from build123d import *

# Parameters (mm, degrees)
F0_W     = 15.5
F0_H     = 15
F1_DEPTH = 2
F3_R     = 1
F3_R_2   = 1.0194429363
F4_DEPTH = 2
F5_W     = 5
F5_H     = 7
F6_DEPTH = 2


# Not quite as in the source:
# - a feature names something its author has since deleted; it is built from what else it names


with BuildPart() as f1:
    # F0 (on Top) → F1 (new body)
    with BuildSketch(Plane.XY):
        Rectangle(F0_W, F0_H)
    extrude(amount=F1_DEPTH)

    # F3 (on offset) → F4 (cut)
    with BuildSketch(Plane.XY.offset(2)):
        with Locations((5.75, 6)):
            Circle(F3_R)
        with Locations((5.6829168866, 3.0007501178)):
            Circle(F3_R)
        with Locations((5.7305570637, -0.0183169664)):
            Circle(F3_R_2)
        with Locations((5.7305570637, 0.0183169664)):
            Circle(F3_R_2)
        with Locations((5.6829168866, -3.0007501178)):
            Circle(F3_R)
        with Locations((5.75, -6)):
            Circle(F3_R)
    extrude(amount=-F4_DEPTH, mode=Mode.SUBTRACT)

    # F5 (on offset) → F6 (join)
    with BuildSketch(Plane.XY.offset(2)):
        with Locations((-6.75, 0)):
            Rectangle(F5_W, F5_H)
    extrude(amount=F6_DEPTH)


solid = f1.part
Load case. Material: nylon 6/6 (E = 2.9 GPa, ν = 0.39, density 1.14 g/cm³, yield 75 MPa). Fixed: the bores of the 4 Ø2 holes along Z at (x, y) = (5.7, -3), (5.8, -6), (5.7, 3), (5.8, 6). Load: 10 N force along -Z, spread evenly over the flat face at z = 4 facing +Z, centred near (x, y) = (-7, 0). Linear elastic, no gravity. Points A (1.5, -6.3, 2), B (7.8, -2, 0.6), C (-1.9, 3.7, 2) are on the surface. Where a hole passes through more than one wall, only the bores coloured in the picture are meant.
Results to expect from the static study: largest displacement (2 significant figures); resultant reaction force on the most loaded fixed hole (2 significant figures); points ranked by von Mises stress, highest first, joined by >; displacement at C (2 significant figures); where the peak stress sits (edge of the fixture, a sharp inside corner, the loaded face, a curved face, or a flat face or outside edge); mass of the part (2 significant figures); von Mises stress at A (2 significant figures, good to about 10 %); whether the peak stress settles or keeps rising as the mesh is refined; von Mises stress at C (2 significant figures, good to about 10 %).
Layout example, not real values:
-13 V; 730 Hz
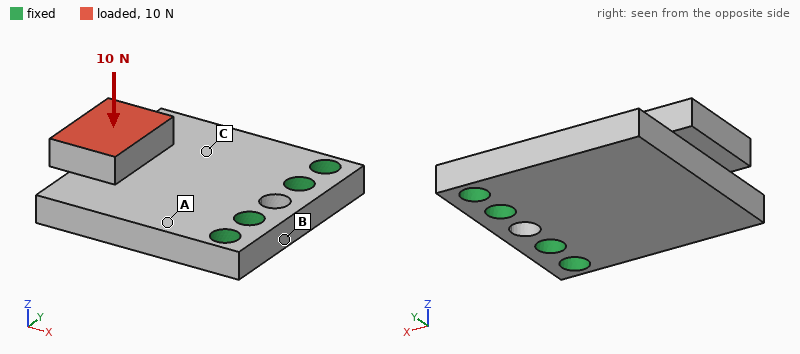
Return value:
0.26 mm; 4.8 N; A > C > B; 0.082 mm; edge of the fixture; 0.57 g; 8.2 MPa; keeps rising; 4.6 MPa
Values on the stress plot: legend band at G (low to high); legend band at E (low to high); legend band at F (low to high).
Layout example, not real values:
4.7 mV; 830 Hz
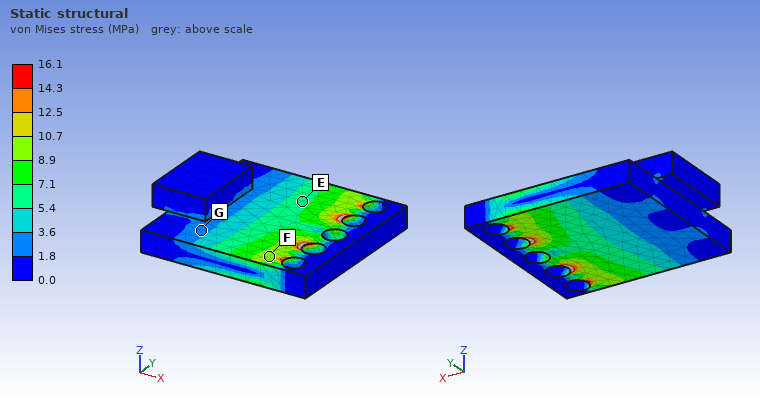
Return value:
1.8 to 3.6 MPa; 5.4 to 7.1 MPa; 8.9 to 10.7 MPa
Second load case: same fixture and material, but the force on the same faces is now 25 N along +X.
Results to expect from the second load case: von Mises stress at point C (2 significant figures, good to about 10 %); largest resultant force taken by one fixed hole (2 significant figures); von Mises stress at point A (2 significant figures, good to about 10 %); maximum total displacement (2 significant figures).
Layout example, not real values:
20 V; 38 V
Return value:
7.8 MPa; 7.6 N; 8.0 MPa; 0.26 mm
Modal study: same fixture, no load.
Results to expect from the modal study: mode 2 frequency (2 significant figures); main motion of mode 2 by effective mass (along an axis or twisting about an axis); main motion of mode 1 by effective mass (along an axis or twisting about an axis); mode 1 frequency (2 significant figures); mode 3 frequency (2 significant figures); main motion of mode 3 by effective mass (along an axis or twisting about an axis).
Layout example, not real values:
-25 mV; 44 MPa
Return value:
6300 Hz; twisting about X; along Z; 2500 Hz; 12 kHz; along Y
